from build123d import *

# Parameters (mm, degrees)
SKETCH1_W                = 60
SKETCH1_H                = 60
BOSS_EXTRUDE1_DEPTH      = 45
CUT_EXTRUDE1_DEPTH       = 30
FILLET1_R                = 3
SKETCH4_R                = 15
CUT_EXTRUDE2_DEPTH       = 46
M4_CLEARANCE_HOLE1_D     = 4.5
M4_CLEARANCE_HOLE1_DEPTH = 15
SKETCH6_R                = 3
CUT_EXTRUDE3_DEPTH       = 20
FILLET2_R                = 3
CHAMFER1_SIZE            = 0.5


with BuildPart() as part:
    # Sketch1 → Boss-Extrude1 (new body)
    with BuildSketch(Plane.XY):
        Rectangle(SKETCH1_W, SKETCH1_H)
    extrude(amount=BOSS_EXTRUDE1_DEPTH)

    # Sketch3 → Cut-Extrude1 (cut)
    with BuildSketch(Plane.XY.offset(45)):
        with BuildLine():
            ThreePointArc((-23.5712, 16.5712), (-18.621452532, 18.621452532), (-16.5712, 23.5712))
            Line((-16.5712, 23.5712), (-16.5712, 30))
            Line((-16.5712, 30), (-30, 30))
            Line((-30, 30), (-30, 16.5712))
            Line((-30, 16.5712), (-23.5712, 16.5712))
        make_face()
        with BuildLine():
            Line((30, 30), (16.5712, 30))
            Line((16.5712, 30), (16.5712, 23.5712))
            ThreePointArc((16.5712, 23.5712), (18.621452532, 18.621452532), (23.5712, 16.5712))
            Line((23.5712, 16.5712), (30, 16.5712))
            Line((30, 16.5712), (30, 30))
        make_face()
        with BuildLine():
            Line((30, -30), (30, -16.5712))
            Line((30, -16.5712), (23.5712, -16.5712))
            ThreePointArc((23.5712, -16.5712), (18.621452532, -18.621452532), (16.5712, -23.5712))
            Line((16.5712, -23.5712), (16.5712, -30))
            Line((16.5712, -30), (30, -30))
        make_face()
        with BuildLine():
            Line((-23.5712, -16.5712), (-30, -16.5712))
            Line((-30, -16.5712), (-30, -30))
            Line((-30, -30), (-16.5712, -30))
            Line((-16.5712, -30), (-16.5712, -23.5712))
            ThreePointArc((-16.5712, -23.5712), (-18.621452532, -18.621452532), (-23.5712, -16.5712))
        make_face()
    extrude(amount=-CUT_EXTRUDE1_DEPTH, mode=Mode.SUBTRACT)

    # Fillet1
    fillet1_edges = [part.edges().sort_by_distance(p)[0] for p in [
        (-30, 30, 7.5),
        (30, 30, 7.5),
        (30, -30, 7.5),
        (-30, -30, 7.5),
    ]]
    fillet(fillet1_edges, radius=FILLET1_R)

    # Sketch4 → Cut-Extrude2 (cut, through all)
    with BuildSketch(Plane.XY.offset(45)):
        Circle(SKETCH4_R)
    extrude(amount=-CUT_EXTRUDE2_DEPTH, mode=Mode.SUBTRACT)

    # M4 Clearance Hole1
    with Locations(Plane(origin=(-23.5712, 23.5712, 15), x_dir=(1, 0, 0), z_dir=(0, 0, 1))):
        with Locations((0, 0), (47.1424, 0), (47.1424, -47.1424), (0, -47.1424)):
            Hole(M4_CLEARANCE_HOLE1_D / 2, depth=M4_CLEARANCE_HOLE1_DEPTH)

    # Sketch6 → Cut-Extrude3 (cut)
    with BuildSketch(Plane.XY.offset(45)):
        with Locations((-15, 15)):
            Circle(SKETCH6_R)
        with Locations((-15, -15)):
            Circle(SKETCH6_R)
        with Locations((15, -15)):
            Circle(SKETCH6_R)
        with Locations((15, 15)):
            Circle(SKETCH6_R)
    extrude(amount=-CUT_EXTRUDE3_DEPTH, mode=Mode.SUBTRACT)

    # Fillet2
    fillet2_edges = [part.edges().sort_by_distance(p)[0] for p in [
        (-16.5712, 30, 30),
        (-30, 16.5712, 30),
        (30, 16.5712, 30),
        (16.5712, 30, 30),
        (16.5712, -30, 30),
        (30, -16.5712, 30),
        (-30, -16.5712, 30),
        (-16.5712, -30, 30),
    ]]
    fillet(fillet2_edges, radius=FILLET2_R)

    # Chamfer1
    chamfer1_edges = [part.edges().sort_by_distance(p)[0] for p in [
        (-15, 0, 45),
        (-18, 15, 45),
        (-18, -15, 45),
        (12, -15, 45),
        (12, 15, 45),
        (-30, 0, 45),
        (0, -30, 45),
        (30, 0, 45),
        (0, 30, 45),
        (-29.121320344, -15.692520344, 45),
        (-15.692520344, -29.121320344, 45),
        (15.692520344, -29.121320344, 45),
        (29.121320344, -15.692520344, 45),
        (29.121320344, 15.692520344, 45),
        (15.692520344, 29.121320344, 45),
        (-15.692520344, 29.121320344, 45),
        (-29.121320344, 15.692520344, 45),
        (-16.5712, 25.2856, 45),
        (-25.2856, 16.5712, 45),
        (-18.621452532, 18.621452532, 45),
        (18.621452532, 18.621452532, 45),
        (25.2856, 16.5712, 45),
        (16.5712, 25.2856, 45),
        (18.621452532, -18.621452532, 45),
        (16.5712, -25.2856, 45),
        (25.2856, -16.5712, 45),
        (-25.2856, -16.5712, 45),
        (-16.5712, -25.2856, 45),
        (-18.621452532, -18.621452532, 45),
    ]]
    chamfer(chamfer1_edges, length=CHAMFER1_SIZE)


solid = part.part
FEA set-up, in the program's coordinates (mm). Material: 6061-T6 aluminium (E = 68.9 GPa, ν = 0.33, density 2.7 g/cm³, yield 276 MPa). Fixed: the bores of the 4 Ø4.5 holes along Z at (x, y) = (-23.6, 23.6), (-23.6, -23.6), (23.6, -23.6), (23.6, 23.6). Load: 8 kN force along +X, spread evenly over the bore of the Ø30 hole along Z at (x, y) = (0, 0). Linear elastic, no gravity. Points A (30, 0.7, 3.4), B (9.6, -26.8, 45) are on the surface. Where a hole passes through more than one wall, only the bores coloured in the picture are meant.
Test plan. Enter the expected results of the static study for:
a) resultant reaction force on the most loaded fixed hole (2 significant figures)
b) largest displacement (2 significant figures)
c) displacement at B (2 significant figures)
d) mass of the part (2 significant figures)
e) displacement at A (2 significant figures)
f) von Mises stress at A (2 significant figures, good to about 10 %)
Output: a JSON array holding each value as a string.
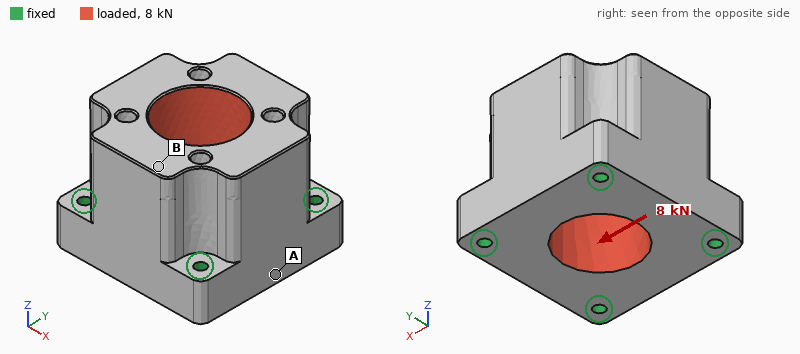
["2.4 kN", "9.1 µm", "7.4 µm", "290 g", "3.5 µm", "5.6 MPa"]
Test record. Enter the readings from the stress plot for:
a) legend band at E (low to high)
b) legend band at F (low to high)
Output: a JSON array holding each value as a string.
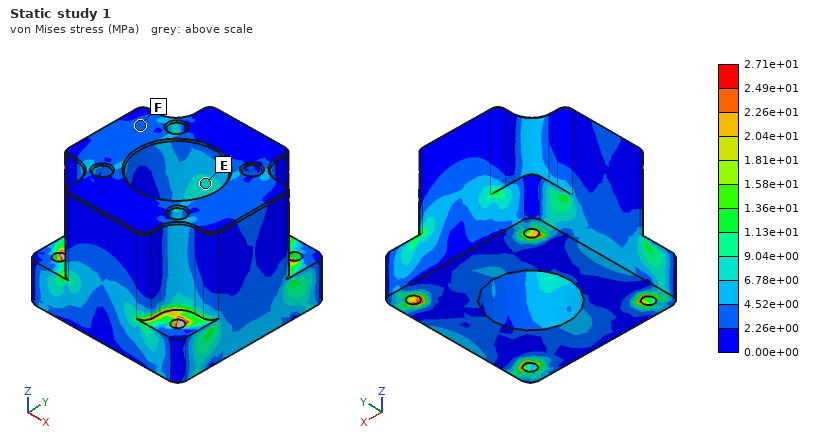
["6.78e+00 to 9.04e+00 MPa", "2.26e+00 to 4.52e+00 MPa"]
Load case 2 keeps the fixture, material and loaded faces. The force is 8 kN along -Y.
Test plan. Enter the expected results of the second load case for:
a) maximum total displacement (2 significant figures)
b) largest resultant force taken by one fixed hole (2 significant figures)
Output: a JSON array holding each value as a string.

["9.1 µm", "2.4 kN"]
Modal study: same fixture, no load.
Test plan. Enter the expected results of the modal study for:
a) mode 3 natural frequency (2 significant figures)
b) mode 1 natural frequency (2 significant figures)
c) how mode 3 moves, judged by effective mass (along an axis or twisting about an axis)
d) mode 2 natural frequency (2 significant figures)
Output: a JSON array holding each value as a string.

["15 kHz", "11 kHz", "along Z", "11 kHz"]
